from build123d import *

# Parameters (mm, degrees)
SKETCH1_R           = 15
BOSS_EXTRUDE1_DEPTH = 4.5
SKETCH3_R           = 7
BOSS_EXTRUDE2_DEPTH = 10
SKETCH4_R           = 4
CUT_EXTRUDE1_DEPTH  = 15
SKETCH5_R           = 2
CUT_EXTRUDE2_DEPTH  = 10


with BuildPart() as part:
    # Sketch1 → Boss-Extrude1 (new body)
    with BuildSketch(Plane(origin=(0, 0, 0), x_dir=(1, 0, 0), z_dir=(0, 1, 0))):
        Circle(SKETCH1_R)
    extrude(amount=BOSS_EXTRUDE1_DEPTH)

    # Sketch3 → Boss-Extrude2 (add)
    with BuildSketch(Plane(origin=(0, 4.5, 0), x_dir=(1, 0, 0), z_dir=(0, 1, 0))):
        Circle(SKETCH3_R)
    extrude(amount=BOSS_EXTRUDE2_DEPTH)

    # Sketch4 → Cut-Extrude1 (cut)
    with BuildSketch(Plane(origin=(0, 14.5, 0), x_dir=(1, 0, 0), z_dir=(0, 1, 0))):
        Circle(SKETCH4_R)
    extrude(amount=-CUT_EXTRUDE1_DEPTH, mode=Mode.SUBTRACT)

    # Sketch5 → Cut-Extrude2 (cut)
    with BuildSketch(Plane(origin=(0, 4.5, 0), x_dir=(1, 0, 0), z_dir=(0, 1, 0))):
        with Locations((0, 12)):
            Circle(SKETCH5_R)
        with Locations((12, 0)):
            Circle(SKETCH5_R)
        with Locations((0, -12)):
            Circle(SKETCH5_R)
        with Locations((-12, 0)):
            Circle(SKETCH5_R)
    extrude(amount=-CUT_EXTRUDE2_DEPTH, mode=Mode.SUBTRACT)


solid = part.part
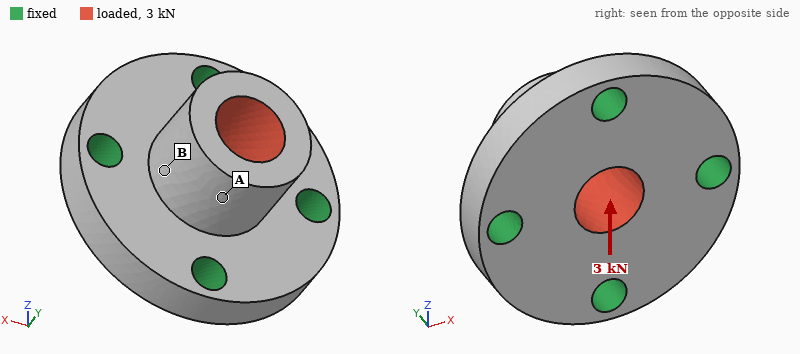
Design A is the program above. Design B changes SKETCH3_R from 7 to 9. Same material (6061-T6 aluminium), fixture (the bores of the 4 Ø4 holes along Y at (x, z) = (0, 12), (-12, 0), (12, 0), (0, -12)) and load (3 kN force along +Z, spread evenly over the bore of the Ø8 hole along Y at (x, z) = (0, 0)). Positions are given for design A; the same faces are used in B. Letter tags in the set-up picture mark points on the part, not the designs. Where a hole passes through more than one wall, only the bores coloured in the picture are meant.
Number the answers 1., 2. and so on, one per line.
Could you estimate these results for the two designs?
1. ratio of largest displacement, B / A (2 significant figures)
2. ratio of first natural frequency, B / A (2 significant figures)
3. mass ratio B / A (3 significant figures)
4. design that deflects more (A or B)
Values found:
1. 0.46
2. 1.1
3. 1.27
4. A
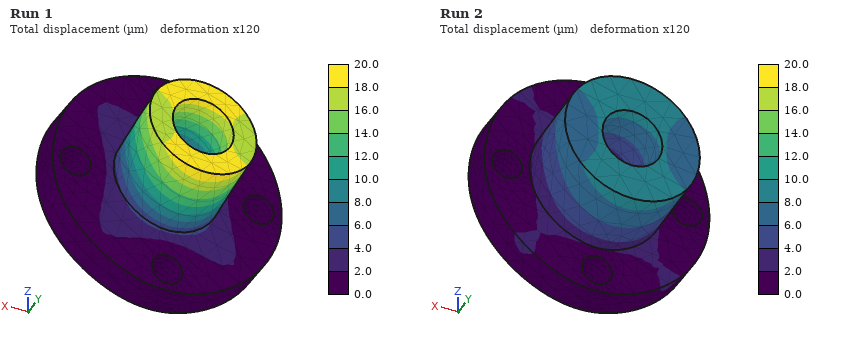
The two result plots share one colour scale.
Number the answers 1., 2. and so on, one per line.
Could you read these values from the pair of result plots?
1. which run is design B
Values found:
1. Run 2
